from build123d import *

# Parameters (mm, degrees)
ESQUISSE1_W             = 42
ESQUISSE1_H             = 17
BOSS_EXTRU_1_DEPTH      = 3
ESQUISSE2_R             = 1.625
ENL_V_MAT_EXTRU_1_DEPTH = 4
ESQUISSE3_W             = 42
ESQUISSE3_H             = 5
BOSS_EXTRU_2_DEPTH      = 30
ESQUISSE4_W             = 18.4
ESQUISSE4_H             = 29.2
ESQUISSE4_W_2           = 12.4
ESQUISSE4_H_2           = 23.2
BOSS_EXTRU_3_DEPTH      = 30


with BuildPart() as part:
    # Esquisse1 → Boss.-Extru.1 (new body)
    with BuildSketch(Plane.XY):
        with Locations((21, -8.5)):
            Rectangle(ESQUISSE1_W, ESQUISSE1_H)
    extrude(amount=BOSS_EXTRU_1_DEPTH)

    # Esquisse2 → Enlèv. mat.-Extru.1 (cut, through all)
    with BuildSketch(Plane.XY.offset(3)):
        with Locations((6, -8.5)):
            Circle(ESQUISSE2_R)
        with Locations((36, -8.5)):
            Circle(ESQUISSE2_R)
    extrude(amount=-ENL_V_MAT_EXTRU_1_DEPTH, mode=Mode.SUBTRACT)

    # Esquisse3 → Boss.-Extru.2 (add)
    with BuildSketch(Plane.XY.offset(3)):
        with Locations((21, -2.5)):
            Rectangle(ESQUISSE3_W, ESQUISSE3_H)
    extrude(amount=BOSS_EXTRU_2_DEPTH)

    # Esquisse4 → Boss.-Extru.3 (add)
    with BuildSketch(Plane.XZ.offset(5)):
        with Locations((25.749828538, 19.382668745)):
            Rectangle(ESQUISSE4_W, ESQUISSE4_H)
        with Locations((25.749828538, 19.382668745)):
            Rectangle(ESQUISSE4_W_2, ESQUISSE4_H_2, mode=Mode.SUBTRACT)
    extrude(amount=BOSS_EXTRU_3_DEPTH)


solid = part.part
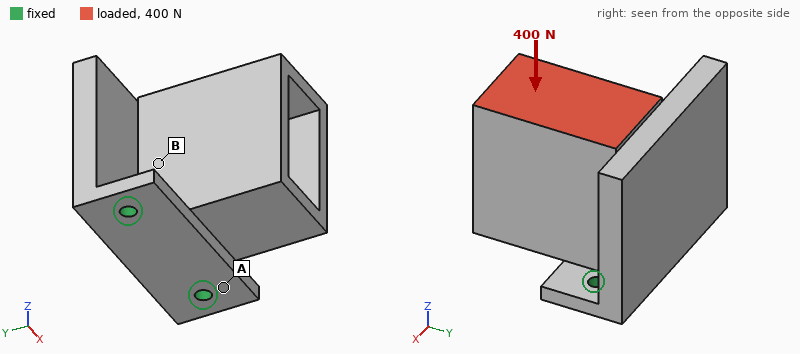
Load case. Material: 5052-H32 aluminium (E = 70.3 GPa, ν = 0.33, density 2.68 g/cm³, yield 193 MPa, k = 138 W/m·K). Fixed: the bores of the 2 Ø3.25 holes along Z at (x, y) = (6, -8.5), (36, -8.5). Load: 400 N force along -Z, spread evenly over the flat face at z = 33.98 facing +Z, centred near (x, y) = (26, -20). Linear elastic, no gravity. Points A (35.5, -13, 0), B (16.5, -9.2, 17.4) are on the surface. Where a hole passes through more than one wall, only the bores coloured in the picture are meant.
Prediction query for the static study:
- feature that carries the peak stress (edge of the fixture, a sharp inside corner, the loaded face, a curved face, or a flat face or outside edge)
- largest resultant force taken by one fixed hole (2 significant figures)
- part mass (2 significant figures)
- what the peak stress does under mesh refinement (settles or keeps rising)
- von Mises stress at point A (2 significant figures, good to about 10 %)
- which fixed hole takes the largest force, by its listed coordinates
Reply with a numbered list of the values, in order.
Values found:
1. edge of the fixture
2. 260 N
3. 43 g
4. keeps rising
5. 29 MPa
6. (36, -8.5)
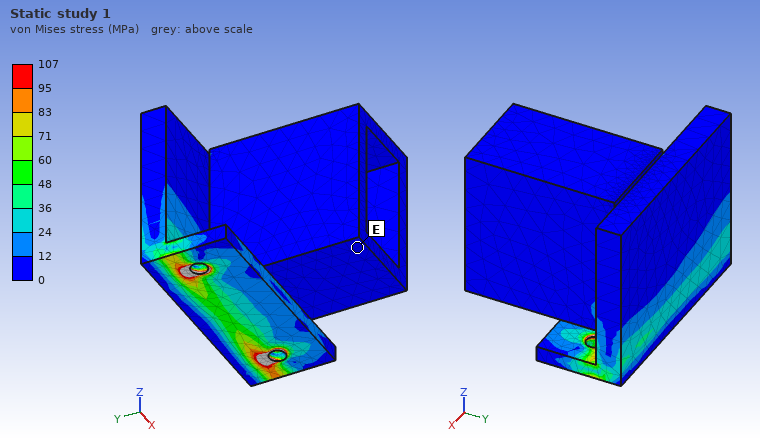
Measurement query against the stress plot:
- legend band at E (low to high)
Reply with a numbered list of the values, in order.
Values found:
1. 0 to 12 MPa
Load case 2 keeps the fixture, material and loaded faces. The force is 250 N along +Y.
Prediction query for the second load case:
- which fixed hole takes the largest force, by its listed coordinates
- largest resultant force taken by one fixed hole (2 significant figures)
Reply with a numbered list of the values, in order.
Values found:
1. (36, -8.5)
2. 160 N
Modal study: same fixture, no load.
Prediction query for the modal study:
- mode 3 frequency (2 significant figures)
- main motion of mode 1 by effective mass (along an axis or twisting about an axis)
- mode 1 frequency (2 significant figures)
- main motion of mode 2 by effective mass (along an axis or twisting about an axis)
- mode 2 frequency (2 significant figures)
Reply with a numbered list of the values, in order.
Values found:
1. 7200 Hz
2. along Y
3. 1100 Hz
4. along X
5. 3500 Hz
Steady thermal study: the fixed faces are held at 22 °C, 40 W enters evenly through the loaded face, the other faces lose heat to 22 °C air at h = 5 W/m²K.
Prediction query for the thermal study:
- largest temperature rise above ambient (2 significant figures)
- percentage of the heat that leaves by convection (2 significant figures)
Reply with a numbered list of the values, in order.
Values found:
1. 68 K
2. 4.1 %
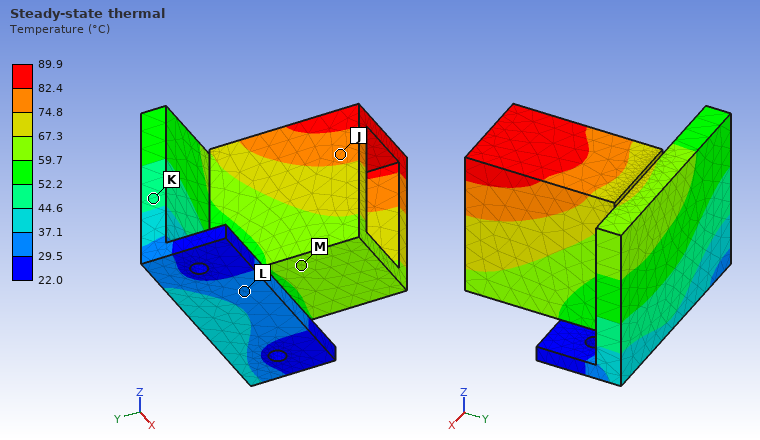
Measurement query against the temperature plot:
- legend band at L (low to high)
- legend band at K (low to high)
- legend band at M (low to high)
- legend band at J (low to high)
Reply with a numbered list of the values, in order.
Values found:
1. 29.5 to 37.1 °C
2. 44.6 to 52.2 °C
3. 59.7 to 67.3 °C
4. 74.8 to 82.4 °C
